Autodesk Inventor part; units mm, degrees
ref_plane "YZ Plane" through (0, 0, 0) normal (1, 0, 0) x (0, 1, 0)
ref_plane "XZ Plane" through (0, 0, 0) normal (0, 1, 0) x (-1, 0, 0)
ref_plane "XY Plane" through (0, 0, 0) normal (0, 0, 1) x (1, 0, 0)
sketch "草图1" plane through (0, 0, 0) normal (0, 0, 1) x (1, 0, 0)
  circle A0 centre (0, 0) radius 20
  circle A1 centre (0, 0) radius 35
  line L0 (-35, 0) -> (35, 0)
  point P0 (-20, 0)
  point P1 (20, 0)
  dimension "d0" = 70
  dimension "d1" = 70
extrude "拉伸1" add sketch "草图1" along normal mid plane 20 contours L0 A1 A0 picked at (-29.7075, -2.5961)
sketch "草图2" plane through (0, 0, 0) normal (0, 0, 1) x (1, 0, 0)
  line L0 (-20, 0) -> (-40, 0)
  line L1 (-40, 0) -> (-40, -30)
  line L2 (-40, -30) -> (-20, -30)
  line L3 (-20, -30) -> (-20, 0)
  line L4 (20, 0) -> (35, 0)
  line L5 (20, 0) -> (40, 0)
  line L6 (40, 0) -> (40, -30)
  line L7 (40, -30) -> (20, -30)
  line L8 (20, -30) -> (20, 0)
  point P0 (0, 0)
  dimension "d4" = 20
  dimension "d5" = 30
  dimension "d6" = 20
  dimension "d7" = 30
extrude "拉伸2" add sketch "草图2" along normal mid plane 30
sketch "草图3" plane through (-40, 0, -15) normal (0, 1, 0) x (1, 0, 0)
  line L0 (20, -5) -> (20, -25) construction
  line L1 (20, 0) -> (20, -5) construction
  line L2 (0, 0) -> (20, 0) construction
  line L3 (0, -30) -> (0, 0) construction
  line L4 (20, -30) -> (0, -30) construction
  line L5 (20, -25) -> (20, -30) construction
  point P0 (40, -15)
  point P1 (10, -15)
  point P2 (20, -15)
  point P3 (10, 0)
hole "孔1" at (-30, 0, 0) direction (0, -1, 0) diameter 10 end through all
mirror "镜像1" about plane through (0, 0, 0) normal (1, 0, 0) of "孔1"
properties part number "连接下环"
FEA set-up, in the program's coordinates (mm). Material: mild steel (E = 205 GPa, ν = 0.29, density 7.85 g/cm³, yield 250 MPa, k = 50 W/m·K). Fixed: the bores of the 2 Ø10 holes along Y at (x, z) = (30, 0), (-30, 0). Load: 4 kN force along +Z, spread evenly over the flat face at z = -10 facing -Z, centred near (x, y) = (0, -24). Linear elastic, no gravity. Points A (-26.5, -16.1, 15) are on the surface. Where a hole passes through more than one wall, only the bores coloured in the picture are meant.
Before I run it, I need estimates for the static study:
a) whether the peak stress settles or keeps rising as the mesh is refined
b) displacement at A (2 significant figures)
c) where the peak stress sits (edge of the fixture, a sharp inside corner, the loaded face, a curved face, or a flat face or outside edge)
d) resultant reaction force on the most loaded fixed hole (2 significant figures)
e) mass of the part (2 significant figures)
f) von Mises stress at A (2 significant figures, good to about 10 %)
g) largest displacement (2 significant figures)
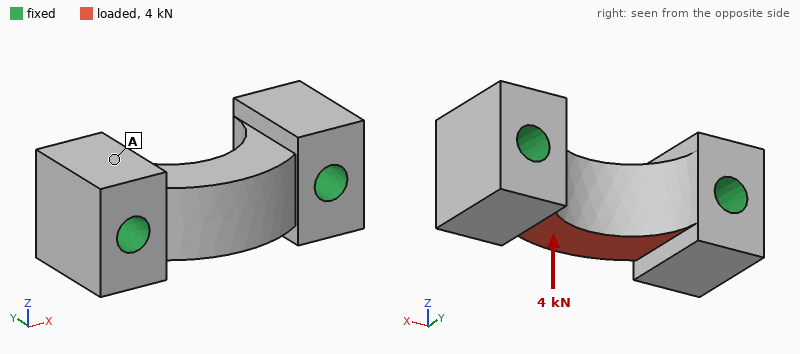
keeps rising
0.54 µm
edge of the fixture
2.0 kN
350 g
3.9 MPa
3.4 µm
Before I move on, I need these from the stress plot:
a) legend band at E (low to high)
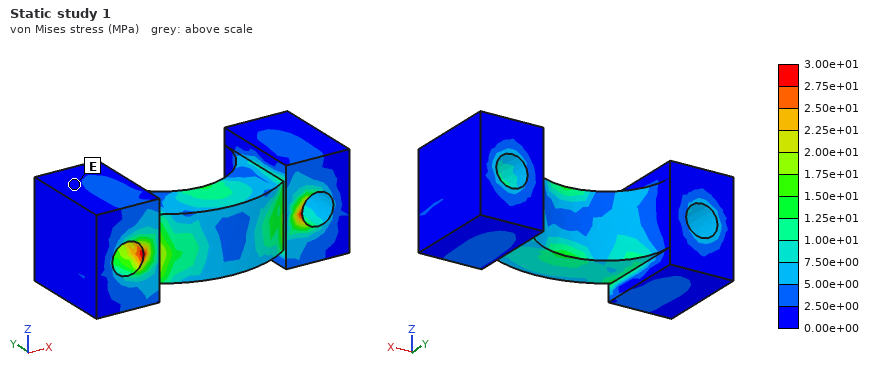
0.00e+00 to 2.50e+00 MPa
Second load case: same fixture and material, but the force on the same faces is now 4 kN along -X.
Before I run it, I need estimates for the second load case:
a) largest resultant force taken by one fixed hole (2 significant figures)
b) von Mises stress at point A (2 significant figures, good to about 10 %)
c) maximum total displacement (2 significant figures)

2.1 kN
1.1 MPa
1.1 µm
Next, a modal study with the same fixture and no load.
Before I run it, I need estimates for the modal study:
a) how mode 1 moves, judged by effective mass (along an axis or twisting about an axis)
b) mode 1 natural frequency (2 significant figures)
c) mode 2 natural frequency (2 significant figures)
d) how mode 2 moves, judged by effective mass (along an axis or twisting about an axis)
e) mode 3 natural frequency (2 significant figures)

along Z
20 kHz
27 kHz
along Y
34 kHz
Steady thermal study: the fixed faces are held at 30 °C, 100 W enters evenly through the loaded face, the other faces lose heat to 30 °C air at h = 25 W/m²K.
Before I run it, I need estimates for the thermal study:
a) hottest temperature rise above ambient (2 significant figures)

63 K
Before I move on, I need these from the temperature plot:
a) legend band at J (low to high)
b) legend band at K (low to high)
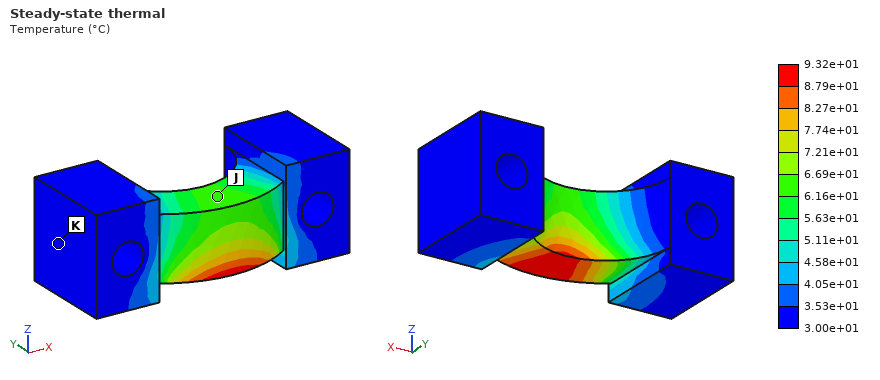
6.16e+01 to 6.69e+01 °C
3.00e+01 to 3.53e+01 °C
